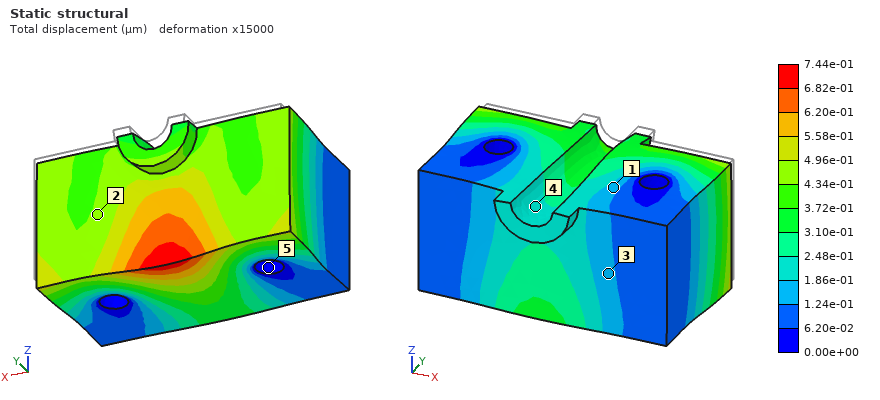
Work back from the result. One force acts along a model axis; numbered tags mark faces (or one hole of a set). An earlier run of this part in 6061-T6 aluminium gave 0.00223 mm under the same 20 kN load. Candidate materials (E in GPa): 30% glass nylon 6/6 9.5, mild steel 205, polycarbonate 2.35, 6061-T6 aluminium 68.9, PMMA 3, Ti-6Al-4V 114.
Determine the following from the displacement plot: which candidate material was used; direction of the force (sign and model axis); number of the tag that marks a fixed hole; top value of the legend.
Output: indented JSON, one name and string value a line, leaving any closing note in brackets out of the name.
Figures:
{
  "which candidate material was used": "mild steel",
  "direction of the force": "-Y",
  "number of the tag that marks a fixed hole": "5",
  "top value of the legend": "7.44e-01 µm"
}
